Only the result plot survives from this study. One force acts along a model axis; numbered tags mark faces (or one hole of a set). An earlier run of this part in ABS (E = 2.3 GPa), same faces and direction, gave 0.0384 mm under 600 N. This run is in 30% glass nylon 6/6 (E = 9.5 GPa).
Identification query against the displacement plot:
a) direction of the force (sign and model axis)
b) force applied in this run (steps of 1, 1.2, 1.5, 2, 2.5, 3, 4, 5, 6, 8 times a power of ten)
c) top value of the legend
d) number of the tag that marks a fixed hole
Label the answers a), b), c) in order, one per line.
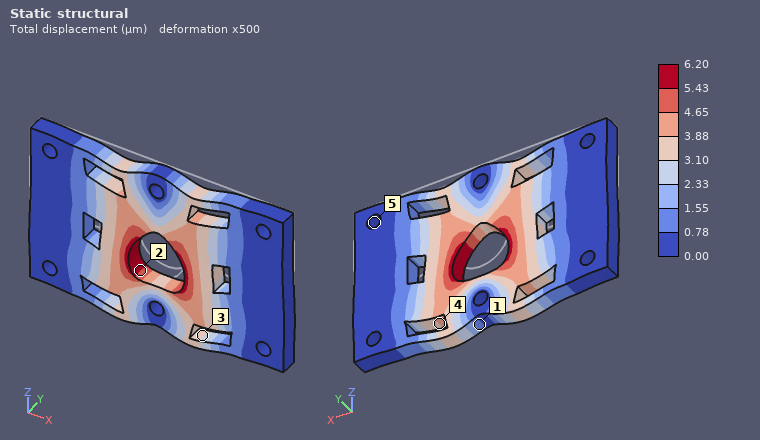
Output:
a) -Z
b) 400 N
c) 6.20 µm
d) 5
